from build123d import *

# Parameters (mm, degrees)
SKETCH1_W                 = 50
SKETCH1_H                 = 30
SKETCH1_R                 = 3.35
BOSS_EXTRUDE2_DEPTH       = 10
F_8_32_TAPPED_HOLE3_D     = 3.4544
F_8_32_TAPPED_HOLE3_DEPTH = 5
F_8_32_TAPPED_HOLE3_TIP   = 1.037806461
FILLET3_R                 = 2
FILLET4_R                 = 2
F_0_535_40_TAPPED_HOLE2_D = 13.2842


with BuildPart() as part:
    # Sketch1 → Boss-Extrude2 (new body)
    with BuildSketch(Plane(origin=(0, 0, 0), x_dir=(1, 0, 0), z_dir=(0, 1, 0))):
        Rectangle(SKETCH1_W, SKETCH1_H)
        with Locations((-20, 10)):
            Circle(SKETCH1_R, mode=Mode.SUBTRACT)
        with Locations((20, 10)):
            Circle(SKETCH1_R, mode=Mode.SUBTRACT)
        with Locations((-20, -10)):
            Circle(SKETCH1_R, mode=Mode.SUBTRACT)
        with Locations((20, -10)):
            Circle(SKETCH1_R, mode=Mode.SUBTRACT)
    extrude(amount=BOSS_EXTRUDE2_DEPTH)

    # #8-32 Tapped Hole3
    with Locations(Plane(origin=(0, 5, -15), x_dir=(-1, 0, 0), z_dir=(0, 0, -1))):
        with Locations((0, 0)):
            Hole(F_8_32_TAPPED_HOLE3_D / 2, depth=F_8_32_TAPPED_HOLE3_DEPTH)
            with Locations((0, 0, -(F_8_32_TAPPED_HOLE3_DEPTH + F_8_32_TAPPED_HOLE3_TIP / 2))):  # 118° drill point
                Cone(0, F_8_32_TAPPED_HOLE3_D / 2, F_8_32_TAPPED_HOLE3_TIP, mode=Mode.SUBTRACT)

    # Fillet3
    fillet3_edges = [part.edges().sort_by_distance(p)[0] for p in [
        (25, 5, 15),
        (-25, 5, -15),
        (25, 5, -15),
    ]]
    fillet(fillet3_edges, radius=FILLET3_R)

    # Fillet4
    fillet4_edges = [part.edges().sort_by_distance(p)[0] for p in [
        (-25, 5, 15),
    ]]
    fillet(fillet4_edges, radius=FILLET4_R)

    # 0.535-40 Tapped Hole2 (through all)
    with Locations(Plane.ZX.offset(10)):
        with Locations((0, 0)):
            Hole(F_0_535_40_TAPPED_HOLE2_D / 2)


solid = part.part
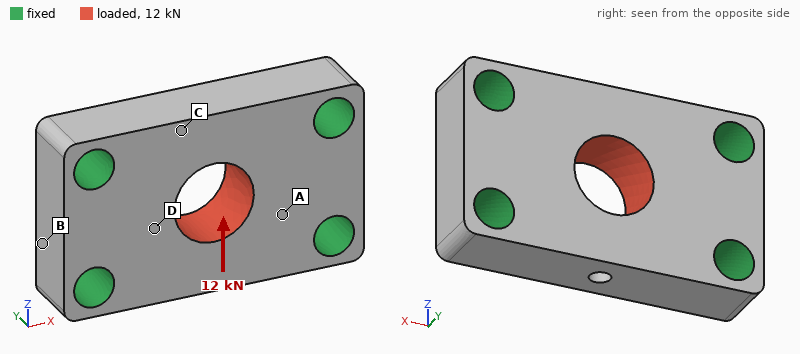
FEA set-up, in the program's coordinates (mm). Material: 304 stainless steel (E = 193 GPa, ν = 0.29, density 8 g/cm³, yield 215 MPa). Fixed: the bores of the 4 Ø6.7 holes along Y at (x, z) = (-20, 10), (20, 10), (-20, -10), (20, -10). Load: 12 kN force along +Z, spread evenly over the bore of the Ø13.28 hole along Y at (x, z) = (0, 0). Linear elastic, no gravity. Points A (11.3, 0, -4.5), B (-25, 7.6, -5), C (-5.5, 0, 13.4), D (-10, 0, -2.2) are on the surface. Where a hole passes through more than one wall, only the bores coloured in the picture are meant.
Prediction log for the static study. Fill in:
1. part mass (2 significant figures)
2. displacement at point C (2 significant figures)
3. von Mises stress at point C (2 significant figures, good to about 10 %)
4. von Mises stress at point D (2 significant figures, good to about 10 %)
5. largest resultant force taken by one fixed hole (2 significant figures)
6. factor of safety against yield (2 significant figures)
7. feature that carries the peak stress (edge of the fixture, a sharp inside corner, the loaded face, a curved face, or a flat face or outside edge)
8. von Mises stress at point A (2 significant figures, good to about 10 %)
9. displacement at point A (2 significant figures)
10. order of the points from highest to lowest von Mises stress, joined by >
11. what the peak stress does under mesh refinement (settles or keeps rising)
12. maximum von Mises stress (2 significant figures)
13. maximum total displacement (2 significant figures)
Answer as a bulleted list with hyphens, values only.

- 97 g
- 4.4 µm
- 23 MPa
- 54 MPa
- 3.8 kN
- 1.9
- a curved face
- 45 MPa
- 2.3 µm
- D > A > C > B
- settles
- 110 MPa
- 6.2 µm
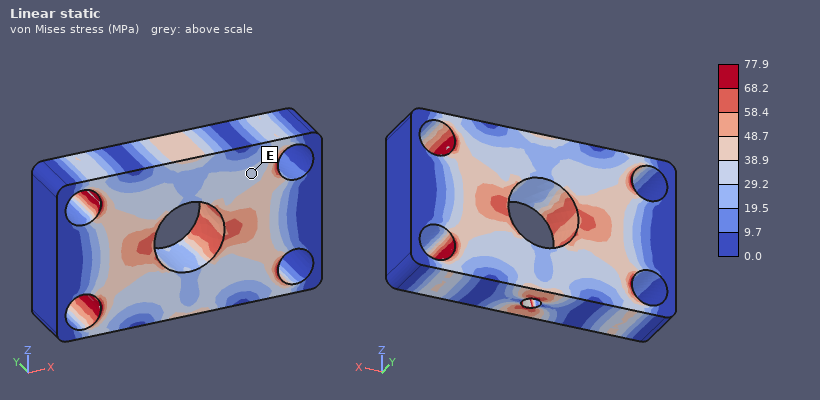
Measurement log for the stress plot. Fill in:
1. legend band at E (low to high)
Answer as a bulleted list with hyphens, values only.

- 29.2 to 38.9 MPa
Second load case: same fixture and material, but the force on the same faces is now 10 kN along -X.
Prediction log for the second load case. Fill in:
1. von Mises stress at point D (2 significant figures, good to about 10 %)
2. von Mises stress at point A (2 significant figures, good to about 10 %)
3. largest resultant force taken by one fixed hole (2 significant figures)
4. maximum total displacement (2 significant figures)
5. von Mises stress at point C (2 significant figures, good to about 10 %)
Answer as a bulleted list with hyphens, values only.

- 22 MPa
- 22 MPa
- 2.6 kN
- 1.9 µm
- 5.1 MPa
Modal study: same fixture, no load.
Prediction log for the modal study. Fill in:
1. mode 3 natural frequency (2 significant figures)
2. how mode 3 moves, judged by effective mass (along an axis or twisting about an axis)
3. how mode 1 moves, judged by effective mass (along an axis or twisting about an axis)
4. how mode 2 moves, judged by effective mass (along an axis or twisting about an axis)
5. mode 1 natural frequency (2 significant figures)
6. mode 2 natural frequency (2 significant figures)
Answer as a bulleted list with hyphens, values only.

- 41 kHz
- along Z
- along Y
- twisting about X
- 29 kHz
- 33 kHz
